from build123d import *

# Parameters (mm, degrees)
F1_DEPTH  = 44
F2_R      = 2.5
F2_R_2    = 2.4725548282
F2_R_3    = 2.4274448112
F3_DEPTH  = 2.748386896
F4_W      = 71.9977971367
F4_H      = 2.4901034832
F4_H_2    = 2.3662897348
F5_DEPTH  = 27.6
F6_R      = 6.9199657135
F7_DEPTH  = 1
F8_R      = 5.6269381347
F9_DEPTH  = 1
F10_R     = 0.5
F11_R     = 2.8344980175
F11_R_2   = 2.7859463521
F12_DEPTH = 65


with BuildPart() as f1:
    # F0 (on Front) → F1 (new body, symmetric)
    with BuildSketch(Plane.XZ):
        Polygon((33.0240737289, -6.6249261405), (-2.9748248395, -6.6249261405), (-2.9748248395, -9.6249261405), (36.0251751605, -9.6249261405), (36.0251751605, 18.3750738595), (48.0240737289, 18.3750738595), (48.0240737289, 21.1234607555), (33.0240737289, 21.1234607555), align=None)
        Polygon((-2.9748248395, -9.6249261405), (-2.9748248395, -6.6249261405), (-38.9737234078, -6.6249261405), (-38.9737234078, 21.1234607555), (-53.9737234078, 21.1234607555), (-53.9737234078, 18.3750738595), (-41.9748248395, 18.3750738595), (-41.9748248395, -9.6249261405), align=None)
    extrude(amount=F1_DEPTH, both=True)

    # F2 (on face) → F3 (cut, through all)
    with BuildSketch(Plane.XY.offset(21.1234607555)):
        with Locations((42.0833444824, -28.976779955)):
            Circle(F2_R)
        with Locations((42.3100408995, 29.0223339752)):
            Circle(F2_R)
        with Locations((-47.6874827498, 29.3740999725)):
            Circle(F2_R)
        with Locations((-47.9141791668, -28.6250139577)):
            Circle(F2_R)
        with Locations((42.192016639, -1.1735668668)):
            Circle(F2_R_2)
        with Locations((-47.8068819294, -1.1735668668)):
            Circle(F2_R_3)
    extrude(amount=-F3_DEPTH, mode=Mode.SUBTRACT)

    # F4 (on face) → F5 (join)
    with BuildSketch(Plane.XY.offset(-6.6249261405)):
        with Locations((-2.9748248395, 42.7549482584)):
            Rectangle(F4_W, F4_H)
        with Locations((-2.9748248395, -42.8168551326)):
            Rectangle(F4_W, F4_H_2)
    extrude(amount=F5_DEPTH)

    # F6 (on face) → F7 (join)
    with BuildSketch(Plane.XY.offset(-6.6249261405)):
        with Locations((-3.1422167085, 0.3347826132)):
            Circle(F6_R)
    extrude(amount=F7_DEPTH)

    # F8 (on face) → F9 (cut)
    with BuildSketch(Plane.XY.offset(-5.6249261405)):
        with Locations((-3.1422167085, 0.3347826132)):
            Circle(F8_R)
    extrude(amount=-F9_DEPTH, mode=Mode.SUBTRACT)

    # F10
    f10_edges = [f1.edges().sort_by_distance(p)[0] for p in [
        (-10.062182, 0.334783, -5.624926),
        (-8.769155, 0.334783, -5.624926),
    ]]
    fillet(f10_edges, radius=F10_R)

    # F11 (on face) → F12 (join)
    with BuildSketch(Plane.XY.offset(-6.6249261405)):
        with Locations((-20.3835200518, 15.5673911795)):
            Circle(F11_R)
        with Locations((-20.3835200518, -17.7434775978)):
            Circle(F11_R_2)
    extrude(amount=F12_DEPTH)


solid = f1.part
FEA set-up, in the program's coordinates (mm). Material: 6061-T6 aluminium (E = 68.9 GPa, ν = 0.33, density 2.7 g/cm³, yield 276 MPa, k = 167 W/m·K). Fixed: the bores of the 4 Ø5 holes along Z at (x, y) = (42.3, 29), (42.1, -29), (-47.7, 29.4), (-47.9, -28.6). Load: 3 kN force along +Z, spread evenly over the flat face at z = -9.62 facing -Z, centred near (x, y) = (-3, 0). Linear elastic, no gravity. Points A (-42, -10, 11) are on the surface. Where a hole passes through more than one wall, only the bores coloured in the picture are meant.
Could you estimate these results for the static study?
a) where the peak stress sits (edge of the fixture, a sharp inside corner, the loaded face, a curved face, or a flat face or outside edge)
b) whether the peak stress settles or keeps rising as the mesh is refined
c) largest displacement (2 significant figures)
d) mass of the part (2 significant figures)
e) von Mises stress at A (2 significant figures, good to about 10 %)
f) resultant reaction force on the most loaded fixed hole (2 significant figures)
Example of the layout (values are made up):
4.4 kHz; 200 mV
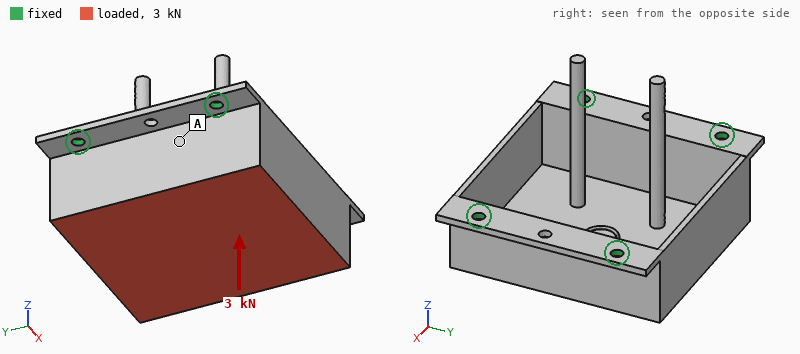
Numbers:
edge of the fixture; keeps rising; 0.44 mm; 140 g; 8.5 MPa; 820 N
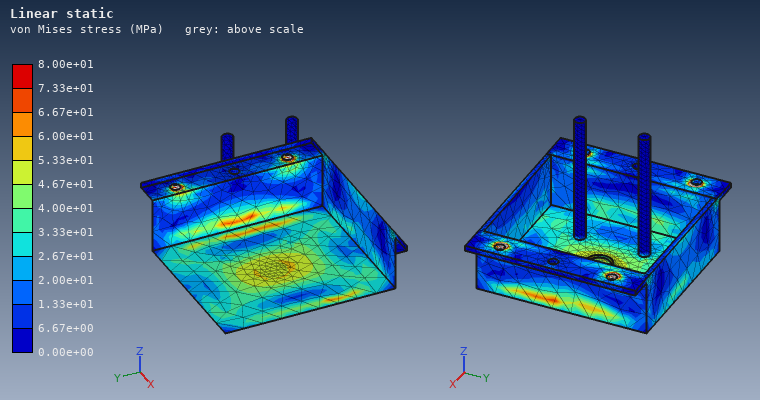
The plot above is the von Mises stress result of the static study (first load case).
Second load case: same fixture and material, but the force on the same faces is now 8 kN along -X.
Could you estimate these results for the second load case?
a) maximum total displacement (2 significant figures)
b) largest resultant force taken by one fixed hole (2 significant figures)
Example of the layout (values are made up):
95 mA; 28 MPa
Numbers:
0.14 mm; 2.8 kN
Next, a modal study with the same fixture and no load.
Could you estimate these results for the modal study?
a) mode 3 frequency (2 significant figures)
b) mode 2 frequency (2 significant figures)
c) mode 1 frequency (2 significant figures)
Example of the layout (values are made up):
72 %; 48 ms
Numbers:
840 Hz; 830 Hz; 810 Hz
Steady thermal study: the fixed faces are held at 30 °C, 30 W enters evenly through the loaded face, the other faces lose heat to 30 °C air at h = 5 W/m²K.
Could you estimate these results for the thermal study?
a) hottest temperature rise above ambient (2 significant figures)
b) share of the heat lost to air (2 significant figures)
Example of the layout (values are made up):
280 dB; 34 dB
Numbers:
17 K; 5.6 %
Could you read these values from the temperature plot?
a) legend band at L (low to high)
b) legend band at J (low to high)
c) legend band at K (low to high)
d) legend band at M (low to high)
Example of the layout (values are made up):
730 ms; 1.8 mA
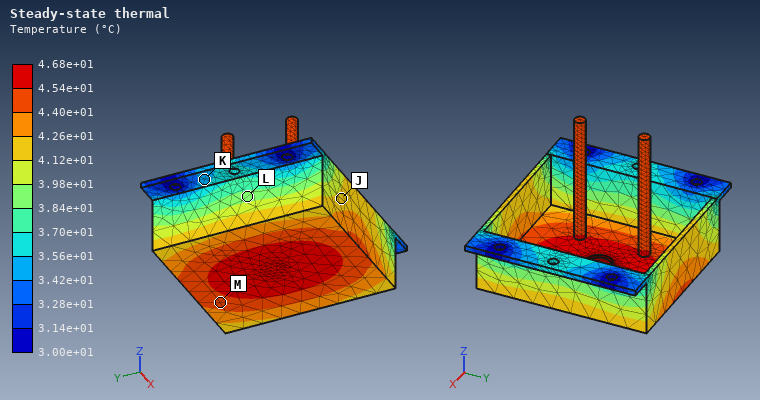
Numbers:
3.84e+01 to 3.98e+01 °C; 4.12e+01 to 4.26e+01 °C; 3.42e+01 to 3.56e+01 °C; 4.40e+01 to 4.54e+01 °C
